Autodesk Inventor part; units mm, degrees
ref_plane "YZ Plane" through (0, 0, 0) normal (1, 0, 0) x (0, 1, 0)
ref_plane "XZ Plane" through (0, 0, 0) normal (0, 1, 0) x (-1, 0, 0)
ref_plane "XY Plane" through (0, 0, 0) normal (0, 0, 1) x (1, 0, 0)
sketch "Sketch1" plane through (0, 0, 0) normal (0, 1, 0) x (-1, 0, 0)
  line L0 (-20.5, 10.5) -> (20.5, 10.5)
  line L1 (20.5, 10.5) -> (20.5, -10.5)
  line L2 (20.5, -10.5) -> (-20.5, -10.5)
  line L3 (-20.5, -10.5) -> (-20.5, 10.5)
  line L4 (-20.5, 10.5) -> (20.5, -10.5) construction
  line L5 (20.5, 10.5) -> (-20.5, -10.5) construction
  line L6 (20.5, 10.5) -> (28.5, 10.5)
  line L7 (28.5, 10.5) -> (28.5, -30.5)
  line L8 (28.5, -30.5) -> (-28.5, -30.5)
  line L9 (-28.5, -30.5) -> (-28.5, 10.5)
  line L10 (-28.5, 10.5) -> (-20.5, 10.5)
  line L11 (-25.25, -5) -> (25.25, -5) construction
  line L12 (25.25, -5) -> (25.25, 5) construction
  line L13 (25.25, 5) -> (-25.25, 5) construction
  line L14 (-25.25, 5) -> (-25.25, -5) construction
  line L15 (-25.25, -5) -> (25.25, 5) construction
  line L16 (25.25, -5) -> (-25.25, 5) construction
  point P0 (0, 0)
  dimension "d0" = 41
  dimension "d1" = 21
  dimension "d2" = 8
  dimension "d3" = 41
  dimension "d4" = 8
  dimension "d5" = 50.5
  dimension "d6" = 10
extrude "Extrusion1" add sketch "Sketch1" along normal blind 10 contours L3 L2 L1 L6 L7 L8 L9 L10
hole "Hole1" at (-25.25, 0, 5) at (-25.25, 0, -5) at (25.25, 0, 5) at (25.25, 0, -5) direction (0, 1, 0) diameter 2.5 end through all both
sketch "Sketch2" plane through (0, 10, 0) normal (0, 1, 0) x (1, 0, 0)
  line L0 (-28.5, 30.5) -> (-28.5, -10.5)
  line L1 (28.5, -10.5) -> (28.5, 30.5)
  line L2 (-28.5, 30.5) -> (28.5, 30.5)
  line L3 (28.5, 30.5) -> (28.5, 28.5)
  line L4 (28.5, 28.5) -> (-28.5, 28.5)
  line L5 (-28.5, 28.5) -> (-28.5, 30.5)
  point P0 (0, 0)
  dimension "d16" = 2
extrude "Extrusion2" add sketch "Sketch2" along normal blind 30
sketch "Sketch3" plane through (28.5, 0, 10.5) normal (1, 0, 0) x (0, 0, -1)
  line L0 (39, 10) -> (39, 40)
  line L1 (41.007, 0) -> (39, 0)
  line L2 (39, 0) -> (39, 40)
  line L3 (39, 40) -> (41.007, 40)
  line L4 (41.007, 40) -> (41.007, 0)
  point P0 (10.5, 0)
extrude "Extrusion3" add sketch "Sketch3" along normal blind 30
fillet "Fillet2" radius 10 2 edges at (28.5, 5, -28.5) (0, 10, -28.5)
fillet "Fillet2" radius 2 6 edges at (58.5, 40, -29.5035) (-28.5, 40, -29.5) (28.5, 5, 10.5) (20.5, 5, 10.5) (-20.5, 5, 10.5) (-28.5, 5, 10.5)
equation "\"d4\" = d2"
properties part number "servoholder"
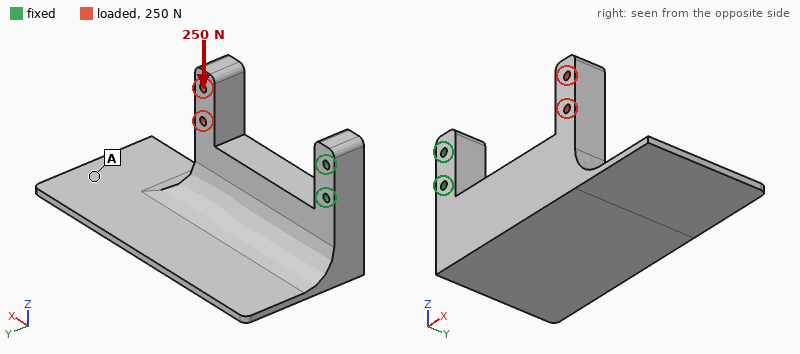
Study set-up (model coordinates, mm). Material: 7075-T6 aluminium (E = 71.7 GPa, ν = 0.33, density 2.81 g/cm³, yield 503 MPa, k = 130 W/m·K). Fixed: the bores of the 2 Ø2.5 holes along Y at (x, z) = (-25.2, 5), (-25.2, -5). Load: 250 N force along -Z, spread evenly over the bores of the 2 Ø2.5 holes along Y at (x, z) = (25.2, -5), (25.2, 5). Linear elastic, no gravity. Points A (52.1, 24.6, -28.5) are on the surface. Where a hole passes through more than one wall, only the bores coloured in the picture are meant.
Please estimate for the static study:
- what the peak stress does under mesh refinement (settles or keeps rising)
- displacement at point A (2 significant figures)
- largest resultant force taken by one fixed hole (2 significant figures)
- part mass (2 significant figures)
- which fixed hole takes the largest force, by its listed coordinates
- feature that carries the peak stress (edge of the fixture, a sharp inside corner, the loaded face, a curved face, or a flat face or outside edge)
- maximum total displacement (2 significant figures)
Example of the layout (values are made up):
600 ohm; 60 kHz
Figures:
keeps rising; 0.41 mm; 800 N; 62 g; (-25.2, 5); edge of the fixture; 0.45 mm
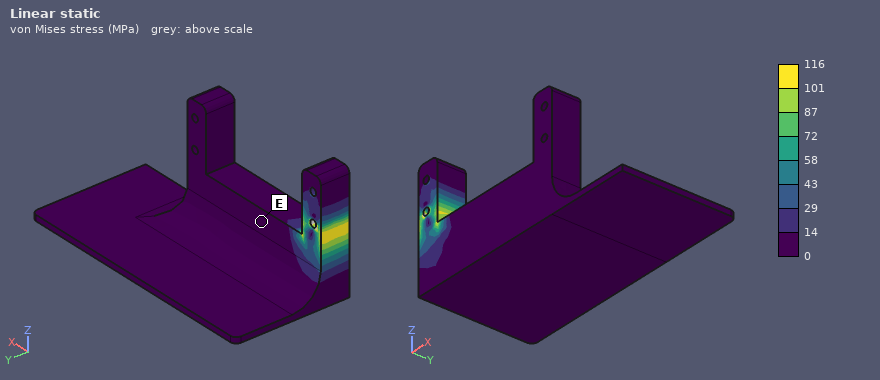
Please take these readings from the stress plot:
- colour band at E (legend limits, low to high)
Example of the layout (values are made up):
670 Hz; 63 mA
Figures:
0 to 14 MPa
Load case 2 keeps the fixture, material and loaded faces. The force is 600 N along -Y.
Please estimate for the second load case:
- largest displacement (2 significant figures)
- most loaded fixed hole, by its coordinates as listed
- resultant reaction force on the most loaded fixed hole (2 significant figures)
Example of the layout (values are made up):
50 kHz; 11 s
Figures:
1.1 mm; (-25.2, -5); 420 N
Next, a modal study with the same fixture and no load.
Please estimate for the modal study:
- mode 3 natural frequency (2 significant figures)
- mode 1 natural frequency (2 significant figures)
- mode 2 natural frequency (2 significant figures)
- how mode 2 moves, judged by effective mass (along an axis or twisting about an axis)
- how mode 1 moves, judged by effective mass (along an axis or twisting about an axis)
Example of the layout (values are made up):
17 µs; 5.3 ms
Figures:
1900 Hz; 760 Hz; 810 Hz; along Y; along Z
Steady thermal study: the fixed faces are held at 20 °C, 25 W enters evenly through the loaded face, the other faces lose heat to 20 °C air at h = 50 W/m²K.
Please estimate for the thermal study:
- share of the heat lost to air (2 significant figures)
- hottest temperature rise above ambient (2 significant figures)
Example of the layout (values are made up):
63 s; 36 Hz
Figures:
51 %; 72 K
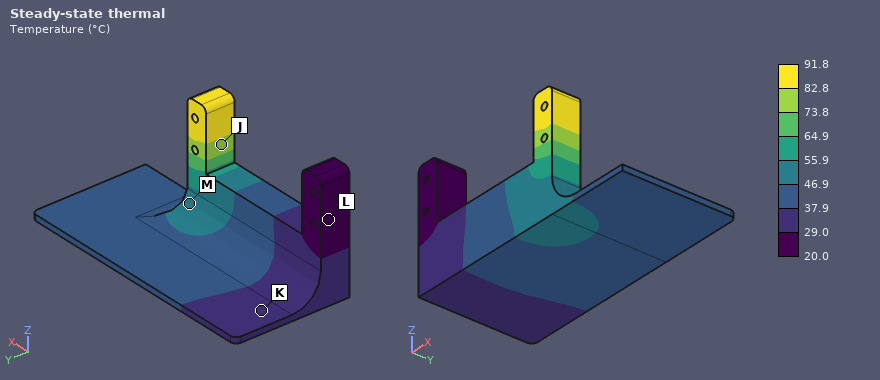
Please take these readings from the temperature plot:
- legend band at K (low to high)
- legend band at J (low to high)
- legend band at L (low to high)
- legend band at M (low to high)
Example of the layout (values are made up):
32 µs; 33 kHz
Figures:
29.0 to 37.9 °C; 73.8 to 82.8 °C; 20.0 to 29.0 °C; 46.9 to 55.9 °C
